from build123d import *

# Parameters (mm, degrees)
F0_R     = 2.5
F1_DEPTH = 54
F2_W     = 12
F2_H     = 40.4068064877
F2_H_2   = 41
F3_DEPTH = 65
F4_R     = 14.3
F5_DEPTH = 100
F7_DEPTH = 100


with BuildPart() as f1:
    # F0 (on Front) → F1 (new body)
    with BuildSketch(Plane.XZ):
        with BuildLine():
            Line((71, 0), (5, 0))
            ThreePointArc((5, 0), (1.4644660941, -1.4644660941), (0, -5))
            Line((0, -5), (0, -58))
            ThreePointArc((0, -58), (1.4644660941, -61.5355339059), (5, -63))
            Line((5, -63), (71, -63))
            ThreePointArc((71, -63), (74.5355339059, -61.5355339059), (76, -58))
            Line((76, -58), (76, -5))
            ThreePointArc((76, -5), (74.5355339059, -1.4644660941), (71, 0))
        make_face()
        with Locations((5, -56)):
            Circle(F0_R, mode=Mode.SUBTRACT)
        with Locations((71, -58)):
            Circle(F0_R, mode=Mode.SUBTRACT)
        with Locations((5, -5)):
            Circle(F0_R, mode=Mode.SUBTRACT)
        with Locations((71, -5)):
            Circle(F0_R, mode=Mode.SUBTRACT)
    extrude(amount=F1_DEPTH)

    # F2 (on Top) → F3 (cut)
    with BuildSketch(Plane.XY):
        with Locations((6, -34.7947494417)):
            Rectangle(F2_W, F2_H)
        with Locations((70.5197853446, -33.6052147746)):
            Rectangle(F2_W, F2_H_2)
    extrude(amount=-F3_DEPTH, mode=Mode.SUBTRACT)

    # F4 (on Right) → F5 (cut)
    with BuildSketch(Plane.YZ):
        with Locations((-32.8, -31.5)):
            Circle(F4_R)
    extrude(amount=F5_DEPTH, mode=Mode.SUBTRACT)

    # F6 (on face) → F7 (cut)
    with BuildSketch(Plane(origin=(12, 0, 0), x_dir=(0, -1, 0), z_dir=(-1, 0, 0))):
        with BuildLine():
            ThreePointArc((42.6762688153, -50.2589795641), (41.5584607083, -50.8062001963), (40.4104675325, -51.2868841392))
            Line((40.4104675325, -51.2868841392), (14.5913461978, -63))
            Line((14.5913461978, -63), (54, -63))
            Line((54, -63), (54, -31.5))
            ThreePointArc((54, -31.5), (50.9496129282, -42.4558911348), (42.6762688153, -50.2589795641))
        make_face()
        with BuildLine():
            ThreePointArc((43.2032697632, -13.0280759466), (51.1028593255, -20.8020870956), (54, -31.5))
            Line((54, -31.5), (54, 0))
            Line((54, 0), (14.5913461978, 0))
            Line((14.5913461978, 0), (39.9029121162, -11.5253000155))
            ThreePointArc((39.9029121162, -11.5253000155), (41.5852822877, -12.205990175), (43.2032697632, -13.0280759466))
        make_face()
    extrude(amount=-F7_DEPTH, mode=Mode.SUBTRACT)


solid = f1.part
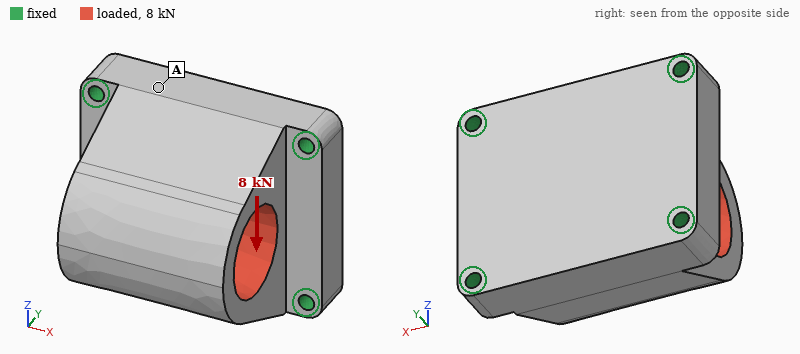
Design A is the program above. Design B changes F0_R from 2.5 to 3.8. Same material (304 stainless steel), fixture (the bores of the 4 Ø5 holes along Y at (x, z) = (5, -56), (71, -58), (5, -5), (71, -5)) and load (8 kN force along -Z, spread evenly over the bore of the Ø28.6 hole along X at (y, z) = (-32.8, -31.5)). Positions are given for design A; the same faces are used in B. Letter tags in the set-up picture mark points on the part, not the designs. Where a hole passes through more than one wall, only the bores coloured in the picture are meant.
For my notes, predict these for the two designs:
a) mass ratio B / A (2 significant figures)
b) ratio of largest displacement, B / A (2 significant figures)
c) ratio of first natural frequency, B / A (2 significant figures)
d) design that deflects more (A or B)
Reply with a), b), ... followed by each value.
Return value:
a) 0.99
b) 0.91
c) 1.1
d) A
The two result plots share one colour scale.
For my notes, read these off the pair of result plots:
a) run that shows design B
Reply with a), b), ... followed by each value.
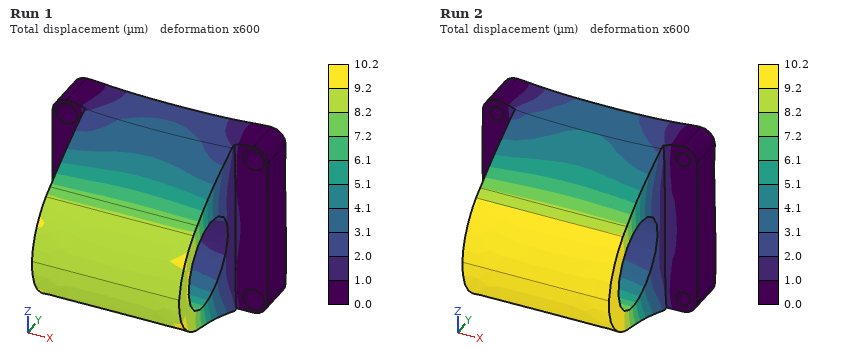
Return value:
a) Run 1
